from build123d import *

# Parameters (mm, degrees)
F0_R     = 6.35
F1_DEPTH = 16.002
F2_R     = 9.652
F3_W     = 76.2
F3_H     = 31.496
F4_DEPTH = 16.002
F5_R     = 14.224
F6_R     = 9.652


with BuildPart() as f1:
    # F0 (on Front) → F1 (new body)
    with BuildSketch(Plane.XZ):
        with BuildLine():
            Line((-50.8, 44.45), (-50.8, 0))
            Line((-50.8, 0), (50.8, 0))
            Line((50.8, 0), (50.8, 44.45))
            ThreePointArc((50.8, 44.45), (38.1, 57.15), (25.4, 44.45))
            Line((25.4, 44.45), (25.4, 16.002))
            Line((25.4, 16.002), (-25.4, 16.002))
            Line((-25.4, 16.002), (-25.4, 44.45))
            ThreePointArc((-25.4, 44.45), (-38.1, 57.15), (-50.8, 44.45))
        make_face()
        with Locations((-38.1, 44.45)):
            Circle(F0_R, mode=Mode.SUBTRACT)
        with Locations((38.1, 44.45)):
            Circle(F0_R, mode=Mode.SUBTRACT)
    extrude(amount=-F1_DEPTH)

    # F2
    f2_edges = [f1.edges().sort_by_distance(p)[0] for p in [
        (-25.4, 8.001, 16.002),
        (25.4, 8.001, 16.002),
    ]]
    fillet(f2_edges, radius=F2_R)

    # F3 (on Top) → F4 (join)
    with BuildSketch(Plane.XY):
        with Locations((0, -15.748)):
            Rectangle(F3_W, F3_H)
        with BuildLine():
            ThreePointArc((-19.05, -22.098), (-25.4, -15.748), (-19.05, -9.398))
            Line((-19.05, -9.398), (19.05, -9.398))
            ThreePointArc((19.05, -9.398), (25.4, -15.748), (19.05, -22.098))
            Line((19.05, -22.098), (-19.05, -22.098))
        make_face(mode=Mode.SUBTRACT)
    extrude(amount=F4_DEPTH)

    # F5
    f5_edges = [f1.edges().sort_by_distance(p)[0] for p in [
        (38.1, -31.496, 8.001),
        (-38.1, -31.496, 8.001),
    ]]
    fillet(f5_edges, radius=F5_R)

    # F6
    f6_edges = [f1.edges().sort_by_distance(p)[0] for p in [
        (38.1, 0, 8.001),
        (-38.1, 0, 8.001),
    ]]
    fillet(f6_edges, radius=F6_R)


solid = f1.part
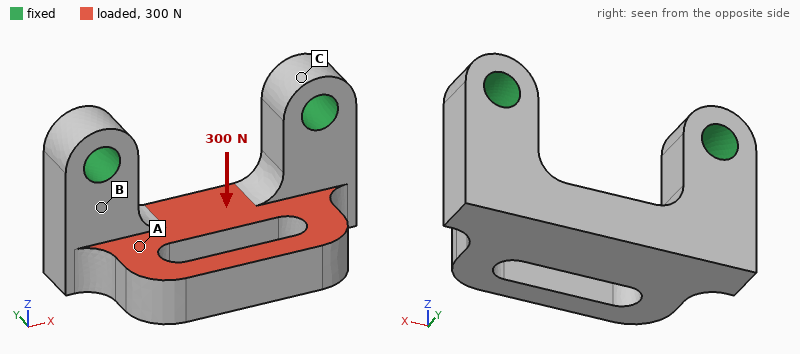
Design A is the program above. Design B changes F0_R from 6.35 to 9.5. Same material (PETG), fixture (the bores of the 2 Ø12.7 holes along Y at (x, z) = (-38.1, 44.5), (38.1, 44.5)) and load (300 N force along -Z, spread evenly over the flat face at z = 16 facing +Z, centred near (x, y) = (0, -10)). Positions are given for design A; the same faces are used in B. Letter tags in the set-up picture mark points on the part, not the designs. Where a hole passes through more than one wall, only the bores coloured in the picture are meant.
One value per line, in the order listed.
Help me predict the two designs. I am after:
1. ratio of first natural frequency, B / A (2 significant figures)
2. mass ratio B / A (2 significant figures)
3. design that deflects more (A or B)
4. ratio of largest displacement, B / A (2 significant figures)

1.1
0.94
A
0.89
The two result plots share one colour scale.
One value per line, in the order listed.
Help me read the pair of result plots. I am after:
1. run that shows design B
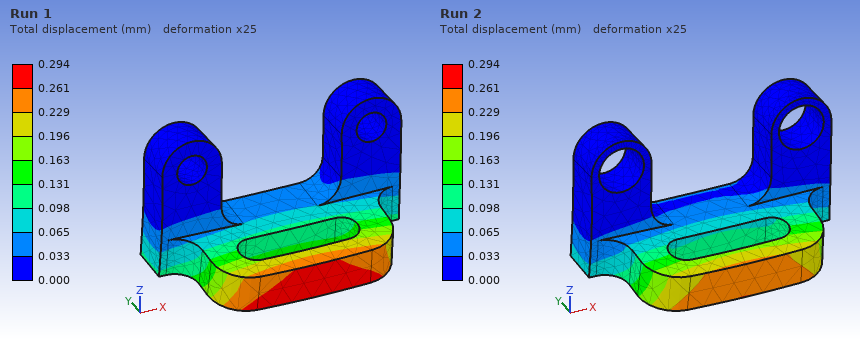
Run 2
